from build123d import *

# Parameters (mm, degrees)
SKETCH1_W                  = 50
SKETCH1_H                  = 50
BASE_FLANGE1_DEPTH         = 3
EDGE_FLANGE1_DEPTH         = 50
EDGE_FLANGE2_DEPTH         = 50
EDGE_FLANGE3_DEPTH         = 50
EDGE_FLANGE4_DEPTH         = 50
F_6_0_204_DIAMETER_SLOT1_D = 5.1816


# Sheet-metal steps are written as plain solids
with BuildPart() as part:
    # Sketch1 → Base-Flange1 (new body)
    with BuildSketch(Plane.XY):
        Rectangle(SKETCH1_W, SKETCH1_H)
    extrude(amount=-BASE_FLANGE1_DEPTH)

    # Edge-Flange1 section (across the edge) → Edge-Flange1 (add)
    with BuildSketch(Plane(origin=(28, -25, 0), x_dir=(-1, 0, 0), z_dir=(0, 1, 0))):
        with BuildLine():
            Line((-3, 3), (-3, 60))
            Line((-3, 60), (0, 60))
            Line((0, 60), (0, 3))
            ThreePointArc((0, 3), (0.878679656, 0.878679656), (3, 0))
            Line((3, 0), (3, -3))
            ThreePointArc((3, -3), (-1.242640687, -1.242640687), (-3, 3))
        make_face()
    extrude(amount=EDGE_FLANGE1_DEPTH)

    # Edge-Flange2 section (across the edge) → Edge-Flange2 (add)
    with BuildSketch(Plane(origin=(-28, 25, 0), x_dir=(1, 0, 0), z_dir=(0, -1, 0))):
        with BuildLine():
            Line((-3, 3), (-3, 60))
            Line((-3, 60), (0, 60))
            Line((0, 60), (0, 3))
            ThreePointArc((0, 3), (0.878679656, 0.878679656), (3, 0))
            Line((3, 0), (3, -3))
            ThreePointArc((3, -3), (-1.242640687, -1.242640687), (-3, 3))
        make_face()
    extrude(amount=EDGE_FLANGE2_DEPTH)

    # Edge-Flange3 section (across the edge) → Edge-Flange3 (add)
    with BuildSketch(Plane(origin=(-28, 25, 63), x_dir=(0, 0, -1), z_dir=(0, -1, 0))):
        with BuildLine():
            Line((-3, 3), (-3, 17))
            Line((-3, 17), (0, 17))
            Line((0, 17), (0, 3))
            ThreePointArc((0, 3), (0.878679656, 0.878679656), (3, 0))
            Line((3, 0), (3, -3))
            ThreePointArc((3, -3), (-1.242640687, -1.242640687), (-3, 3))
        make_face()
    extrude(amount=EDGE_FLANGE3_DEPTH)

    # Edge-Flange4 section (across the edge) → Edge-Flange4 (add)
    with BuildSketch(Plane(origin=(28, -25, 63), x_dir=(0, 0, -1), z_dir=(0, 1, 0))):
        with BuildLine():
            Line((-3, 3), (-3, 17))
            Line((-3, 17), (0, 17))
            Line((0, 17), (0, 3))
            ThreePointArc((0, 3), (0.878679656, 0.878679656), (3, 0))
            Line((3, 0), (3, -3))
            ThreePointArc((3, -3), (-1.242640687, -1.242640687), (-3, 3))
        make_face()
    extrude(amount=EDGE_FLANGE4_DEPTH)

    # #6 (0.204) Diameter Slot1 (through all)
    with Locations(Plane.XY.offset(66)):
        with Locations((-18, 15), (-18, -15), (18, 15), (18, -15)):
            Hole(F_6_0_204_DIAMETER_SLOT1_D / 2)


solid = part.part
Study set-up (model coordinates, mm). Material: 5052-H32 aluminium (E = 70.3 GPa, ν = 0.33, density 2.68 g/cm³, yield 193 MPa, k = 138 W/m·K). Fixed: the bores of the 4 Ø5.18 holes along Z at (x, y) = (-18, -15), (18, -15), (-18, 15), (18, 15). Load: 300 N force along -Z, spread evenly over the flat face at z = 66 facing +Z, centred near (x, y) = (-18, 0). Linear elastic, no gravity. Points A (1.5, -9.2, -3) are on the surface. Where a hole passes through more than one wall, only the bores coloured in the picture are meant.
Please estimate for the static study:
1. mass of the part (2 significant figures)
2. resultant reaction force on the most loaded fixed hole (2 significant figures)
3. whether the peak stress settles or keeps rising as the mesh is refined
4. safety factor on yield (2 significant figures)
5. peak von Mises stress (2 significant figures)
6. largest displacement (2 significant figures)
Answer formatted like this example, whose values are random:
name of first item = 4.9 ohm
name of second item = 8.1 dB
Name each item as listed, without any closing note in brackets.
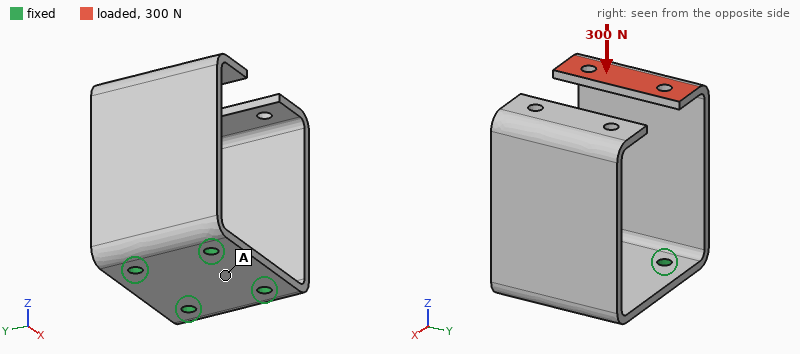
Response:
mass of the part = 87 g
resultant reaction force on the most loaded fixed hole = 150 N
whether the peak stress settles or keeps rising as the mesh is refined = settles
safety factor on yield = 3.5
peak von Mises stress = 55 MPa
largest displacement = 1.2 mm
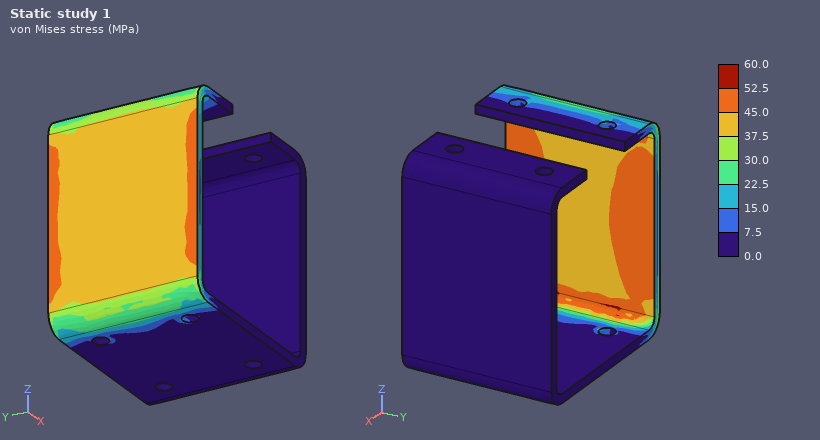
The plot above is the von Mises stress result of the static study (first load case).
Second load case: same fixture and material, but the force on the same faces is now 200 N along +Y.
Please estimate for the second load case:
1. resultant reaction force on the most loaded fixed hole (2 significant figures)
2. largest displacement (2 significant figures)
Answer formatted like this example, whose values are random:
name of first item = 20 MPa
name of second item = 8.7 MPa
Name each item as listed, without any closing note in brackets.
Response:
resultant reaction force on the most loaded fixed hole = 430 N
largest displacement = 0.53 mm
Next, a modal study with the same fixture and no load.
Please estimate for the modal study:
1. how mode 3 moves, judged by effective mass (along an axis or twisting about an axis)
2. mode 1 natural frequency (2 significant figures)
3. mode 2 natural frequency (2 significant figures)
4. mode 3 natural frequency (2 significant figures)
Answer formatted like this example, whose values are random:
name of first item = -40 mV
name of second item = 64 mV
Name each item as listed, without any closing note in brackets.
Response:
how mode 3 moves, judged by effective mass = along Y
mode 1 natural frequency = 340 Hz
mode 2 natural frequency = 340 Hz
mode 3 natural frequency = 1000 Hz
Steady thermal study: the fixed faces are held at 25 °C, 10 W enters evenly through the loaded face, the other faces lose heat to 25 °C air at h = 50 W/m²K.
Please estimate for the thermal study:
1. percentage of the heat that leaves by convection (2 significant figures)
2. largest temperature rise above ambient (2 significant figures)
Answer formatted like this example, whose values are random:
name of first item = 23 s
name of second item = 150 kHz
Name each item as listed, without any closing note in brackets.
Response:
percentage of the heat that leaves by convection = 55 %
largest temperature rise above ambient = 26 K
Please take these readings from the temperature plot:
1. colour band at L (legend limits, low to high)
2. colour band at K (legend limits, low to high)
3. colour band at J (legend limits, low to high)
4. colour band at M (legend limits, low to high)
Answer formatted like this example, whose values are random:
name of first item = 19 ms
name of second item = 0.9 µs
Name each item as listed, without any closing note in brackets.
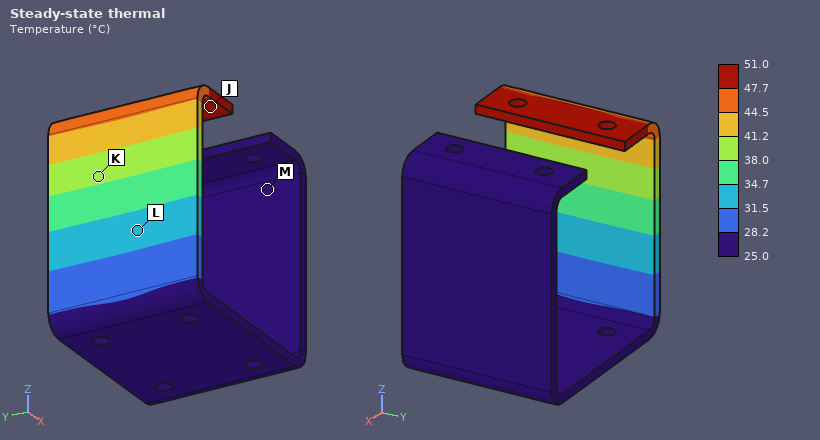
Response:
colour band at L = 31.5 to 34.7 °C
colour band at K = 38.0 to 41.2 °C
colour band at J = 47.7 to 51.0 °C
colour band at M = 25.0 to 28.2 °C
